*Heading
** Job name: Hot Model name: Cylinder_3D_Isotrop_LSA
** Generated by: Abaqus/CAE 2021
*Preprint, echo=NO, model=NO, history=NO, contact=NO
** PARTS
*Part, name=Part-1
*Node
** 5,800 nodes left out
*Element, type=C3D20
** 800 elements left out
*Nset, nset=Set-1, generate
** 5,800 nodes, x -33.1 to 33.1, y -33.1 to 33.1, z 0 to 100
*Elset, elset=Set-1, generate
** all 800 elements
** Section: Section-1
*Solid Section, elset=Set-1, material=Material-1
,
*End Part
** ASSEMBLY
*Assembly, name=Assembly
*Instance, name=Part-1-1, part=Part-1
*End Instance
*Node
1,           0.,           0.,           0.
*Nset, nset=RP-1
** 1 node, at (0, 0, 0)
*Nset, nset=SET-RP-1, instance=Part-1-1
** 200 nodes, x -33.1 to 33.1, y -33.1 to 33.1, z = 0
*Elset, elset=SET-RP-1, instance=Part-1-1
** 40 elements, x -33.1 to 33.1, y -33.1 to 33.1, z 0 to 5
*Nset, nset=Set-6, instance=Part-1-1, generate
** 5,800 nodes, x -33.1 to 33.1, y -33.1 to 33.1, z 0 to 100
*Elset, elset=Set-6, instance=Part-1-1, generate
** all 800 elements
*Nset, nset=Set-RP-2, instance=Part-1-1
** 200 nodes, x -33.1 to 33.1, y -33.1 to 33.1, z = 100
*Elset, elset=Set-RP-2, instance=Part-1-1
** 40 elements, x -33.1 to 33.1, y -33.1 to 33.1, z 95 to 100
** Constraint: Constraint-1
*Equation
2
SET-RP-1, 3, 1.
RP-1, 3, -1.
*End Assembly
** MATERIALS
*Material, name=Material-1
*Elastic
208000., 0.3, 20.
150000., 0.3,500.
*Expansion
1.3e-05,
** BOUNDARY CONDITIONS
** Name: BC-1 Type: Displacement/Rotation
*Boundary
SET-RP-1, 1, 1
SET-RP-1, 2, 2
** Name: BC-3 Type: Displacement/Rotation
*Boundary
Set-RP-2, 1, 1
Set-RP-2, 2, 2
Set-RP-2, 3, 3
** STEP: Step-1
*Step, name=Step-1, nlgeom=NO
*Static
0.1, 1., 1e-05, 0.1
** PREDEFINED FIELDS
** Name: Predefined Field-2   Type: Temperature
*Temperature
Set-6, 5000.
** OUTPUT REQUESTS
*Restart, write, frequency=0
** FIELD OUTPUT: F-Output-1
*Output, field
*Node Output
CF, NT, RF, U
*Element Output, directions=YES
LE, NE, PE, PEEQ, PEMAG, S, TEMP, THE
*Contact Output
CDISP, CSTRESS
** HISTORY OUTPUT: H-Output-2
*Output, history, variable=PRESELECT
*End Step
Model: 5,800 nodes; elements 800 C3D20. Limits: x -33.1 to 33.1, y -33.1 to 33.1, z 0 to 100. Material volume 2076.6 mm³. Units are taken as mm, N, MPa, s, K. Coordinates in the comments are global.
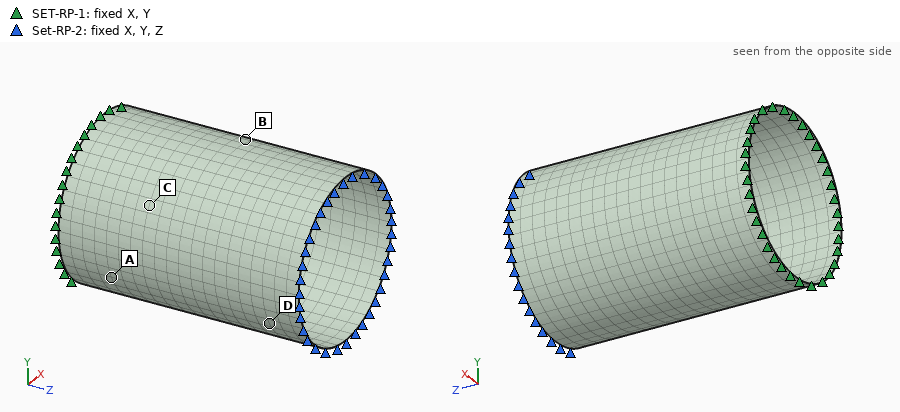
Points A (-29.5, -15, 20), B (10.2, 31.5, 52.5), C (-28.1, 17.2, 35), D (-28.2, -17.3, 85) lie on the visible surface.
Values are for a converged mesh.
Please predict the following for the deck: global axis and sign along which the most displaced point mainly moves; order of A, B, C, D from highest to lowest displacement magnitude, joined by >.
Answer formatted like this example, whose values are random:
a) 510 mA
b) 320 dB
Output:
a) -Z
b) A > C > B > D
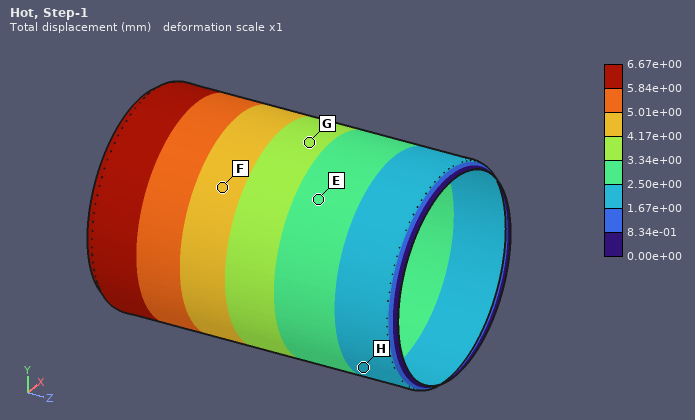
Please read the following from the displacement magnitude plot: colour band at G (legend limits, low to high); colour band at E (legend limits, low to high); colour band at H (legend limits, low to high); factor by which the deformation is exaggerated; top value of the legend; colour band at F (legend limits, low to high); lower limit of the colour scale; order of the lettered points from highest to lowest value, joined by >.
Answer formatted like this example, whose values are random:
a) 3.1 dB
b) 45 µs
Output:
a) 3.34e+00 to 4.17e+00 mm
b) 2.50e+00 to 3.34e+00 mm
c) 1.67e+00 to 2.50e+00 mm
d) 1
e) 6.67e+00 mm
f) 4.17e+00 to 5.01e+00 mm
g) 0.00e+00 mm
h) F > G > E > H
